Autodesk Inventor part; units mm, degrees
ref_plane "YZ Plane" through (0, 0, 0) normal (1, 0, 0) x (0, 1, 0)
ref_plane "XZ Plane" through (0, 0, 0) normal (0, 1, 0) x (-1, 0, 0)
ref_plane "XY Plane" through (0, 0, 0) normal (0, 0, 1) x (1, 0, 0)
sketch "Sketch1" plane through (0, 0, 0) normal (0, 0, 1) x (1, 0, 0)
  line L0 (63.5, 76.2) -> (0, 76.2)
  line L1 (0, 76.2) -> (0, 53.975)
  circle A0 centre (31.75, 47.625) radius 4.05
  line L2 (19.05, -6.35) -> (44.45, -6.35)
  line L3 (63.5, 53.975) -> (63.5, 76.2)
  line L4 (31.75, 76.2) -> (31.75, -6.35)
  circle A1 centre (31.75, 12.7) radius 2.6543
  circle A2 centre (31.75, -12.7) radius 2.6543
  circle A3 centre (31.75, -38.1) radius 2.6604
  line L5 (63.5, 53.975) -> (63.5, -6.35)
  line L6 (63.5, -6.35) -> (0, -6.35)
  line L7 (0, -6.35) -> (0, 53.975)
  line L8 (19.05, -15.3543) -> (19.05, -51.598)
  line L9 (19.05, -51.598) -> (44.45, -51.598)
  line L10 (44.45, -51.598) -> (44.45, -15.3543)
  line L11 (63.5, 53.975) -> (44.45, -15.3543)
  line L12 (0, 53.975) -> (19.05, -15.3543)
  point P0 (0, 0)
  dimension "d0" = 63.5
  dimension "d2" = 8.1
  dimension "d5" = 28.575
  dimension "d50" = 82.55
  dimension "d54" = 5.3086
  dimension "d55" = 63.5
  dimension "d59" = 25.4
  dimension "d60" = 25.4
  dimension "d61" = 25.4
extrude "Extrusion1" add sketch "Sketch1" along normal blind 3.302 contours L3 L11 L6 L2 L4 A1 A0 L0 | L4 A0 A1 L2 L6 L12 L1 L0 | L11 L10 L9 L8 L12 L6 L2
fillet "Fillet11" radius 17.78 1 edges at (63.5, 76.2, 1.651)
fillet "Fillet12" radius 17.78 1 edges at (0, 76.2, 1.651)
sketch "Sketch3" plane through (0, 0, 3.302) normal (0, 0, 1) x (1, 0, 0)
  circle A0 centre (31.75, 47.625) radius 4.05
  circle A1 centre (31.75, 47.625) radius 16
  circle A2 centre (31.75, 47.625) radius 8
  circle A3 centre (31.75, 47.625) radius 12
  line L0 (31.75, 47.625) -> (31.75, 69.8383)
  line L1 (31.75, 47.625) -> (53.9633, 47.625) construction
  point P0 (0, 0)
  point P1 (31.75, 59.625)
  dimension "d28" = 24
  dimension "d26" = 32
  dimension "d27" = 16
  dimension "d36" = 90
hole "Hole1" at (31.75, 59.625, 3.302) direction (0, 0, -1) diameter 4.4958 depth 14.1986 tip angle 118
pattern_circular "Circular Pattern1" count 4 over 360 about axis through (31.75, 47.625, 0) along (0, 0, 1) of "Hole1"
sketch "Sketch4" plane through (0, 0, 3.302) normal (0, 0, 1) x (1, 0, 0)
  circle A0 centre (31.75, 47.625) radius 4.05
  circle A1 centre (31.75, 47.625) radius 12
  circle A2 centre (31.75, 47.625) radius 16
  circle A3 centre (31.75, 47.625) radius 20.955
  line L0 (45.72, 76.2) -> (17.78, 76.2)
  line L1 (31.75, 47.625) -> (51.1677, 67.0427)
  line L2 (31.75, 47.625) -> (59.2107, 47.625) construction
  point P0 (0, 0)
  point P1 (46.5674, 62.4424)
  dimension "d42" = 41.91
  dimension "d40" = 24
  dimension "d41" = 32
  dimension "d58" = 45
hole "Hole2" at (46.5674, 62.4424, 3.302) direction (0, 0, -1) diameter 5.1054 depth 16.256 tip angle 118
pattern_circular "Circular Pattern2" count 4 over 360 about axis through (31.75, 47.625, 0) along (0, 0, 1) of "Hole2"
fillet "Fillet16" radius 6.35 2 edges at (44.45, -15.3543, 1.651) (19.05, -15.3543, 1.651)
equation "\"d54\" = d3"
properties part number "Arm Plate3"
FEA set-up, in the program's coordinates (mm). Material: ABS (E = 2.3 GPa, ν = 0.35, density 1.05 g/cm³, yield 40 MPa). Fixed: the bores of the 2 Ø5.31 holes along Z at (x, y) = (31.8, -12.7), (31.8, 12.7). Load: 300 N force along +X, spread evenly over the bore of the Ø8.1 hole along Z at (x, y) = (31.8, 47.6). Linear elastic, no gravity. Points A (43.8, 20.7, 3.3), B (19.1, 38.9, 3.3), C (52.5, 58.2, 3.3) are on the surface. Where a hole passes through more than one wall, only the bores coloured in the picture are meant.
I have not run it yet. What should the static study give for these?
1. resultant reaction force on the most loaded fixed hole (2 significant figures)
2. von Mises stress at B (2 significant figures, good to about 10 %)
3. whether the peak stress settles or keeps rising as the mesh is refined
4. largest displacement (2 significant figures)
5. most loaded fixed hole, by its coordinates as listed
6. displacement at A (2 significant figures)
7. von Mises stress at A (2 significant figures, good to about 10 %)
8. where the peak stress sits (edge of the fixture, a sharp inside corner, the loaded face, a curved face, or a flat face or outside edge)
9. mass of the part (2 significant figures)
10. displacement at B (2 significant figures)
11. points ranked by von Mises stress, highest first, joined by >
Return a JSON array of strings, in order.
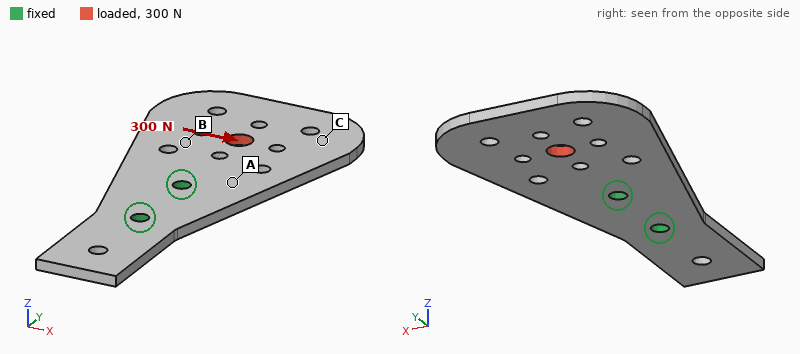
["630 N", "3.6 MPa", "keeps rising", "0.78 mm", "(31.8, 12.7)", "0.14 mm", "6.3 MPa", "edge of the fixture", "17 g", "0.36 mm", "A > B > C"]
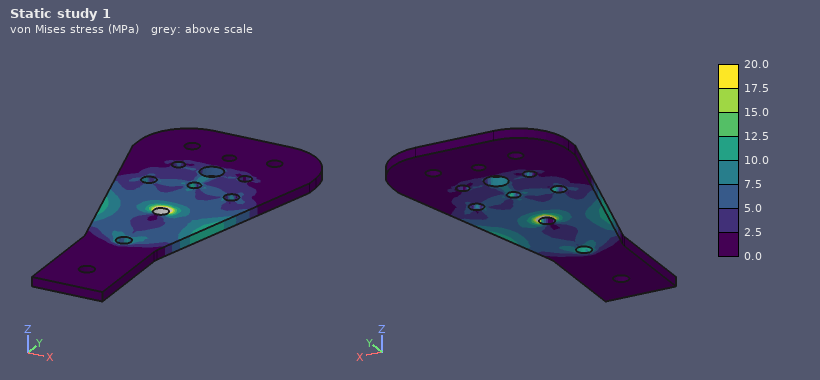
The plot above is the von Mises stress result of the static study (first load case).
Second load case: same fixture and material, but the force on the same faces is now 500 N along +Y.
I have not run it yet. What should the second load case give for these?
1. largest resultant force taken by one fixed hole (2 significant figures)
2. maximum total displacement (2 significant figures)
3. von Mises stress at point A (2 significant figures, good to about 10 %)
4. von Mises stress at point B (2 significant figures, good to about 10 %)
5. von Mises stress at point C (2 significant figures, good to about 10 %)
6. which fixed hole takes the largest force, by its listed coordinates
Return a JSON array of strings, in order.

["370 N", "0.11 mm", "2.7 MPa", "1.9 MPa", "1.2 MPa", "(31.8, 12.7)"]
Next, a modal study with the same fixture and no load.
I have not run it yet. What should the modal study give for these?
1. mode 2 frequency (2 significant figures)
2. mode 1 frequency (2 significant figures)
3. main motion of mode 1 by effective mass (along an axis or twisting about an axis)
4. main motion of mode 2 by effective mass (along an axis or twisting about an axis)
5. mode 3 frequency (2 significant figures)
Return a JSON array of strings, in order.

["360 Hz", "180 Hz", "along Z", "twisting about Y", "560 Hz"]
